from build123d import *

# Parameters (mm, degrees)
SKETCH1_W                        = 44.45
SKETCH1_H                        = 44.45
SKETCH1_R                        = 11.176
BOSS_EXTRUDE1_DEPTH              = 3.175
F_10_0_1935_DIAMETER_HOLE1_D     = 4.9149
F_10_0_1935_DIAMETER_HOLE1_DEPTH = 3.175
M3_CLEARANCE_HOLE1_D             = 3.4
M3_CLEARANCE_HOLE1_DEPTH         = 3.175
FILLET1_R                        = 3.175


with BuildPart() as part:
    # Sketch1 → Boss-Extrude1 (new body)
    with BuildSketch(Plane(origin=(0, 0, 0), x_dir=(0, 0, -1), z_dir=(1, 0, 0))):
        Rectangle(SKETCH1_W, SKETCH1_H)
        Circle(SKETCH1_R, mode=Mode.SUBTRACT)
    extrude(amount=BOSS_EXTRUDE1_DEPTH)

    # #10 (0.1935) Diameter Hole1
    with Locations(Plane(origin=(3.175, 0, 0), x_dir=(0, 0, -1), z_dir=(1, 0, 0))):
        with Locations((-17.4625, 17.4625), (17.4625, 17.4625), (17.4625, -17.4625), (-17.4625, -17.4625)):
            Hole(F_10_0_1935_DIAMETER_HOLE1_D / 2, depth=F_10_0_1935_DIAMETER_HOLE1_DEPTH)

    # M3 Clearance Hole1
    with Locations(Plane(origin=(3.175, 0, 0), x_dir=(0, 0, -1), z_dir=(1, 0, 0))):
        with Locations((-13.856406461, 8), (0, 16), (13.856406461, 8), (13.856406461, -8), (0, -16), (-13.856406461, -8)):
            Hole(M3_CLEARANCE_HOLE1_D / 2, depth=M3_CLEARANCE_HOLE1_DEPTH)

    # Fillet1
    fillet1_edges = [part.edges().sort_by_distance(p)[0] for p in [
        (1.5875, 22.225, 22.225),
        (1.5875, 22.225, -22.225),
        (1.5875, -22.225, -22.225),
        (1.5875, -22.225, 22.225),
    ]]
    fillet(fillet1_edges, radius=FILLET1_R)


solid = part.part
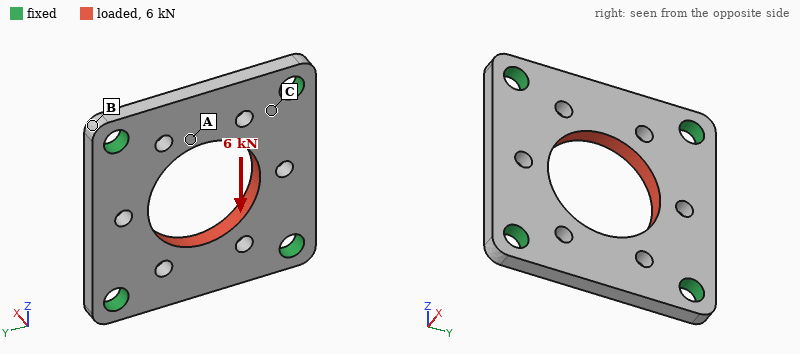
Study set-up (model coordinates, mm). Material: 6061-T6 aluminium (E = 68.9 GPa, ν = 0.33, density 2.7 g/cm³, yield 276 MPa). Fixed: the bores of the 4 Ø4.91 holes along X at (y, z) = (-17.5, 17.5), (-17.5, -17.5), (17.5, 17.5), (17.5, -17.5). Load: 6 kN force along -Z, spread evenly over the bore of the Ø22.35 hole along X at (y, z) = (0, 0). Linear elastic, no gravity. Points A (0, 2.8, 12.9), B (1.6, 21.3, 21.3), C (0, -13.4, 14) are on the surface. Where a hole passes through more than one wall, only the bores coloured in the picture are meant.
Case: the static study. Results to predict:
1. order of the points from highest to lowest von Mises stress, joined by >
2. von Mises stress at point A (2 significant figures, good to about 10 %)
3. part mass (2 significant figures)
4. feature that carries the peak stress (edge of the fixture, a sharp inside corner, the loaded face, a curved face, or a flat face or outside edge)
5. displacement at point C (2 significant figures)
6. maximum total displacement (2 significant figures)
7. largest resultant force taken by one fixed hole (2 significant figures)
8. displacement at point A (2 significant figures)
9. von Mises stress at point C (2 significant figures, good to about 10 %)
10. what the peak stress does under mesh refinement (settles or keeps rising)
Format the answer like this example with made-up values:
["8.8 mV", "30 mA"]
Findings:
["C > A > B", "29 MPa", "12 g", "edge of the fixture", "4.4 µm", "20 µm", "1.6 kN", "18 µm", "56 MPa", "keeps rising"]
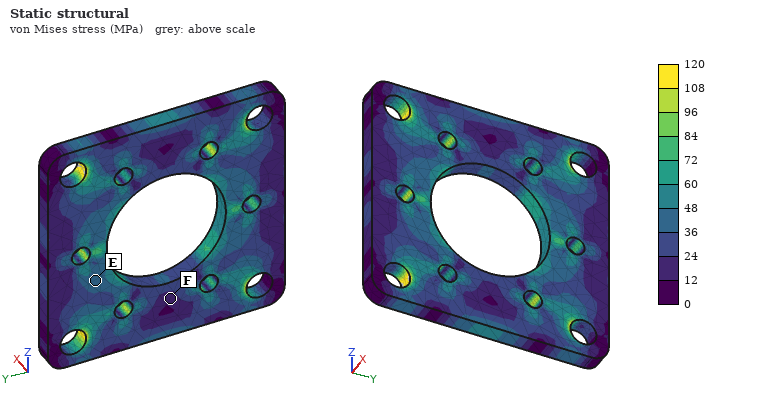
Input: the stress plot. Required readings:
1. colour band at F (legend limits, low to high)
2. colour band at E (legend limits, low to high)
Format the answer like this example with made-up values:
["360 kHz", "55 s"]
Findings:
["12 to 24 MPa", "36 to 48 MPa"]
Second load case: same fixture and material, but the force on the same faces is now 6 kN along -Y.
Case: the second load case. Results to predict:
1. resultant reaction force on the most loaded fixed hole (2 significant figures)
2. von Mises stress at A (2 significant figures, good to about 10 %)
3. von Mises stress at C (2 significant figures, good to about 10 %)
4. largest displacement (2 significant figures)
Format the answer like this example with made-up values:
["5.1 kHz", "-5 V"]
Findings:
["1.6 kN", "45 MPa", "51 MPa", "19 µm"]
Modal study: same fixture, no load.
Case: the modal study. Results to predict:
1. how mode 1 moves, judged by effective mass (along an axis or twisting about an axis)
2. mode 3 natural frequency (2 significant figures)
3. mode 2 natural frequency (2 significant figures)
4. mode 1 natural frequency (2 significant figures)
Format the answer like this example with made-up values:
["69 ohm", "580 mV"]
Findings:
["along X", "16 kHz", "16 kHz", "14 kHz"]
